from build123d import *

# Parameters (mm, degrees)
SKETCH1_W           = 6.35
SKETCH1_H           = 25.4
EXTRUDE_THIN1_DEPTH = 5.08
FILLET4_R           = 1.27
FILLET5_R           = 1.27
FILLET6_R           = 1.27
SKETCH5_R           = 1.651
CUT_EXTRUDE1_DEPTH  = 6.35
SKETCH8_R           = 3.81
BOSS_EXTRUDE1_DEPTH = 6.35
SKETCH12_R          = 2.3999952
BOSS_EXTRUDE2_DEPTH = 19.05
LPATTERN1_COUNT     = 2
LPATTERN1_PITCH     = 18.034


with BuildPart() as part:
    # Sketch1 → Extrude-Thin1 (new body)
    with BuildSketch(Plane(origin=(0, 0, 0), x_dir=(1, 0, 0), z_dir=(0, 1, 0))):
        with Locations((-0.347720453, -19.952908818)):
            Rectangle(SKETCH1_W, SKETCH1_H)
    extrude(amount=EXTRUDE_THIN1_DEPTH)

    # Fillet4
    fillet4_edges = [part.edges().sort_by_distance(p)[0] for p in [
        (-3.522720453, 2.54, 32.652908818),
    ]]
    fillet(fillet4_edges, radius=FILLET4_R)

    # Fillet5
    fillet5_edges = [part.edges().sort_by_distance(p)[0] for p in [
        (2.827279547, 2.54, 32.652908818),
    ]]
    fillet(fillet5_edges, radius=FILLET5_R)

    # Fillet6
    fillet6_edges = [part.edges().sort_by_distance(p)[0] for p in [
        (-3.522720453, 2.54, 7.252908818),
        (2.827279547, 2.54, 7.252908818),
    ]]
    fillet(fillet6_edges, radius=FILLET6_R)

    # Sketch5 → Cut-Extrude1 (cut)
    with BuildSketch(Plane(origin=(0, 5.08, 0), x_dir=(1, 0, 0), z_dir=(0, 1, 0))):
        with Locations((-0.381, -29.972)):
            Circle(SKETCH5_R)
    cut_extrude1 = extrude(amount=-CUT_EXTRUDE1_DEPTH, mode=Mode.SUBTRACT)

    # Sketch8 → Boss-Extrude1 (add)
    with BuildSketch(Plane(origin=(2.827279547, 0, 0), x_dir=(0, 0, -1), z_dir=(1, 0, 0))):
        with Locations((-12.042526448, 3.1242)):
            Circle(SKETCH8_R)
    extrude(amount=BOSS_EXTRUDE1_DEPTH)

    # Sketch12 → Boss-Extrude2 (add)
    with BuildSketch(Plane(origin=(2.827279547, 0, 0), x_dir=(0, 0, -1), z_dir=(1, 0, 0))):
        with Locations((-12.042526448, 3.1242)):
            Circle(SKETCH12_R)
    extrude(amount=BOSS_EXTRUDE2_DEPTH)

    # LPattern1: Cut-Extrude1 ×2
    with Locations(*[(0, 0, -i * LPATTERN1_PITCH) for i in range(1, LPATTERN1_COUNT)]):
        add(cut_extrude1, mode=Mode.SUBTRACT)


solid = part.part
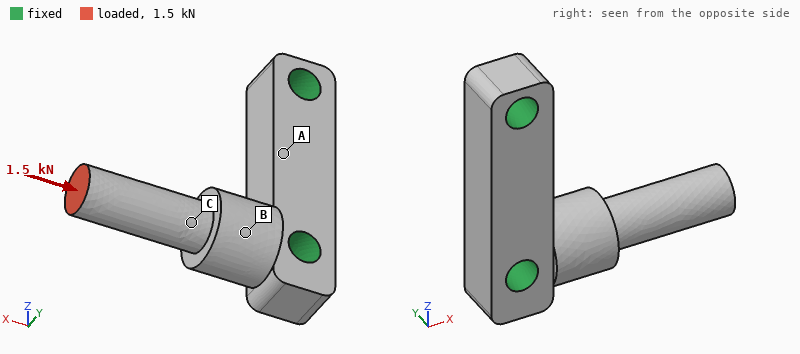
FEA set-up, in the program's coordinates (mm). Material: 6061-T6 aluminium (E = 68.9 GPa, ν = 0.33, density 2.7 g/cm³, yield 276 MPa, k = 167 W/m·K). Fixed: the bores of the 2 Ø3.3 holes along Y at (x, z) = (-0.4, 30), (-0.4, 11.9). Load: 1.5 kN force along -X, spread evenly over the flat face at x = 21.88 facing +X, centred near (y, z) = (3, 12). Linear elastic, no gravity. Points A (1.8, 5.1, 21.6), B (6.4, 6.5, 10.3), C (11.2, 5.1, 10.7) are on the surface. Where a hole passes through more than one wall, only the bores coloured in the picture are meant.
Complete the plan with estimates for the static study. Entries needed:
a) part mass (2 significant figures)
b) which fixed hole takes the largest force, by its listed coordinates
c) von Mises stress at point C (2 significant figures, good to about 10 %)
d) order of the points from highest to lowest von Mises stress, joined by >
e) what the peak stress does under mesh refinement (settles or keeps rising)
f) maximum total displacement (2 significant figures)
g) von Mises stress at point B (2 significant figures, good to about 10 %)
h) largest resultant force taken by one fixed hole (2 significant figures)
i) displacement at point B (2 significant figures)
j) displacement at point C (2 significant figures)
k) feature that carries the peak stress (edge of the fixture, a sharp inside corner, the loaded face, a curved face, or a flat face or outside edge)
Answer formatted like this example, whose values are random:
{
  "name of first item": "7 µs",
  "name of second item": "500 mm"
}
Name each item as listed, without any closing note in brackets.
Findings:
{
  "part mass": "3.4 g",
  "which fixed hole takes the largest force, by its listed coordinates": "(-0.4, 11.9)",
  "von Mises stress at point C": "81 MPa",
  "order of the points from highest to lowest von Mises stress, joined by >": "C > B > A",
  "what the peak stress does under mesh refinement": "keeps rising",
  "maximum total displacement": "25 µm",
  "von Mises stress at point B": "22 MPa",
  "largest resultant force taken by one fixed hole": "1.5 kN",
  "displacement at point B": "6.5 µm",
  "displacement at point C": "11 µm",
  "feature that carries the peak stress": "edge of the fixture"
}
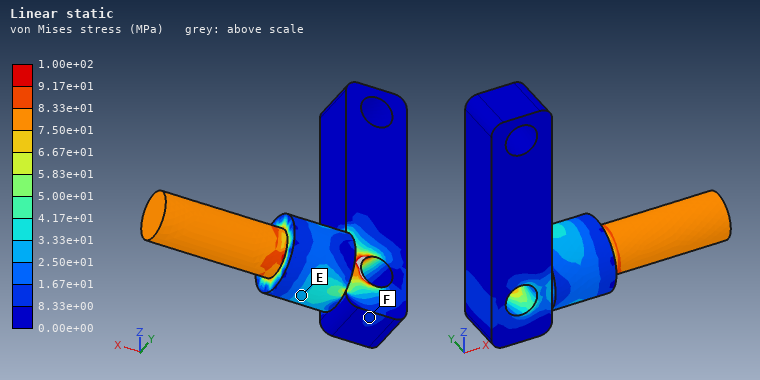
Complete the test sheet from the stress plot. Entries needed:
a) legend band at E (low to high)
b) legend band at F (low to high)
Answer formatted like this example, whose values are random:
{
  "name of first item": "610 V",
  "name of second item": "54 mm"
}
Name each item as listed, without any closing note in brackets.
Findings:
{
  "legend band at E": "2.50e+01 to 3.33e+01 MPa",
  "legend band at F": "8.33e+00 to 1.67e+01 MPa"
}
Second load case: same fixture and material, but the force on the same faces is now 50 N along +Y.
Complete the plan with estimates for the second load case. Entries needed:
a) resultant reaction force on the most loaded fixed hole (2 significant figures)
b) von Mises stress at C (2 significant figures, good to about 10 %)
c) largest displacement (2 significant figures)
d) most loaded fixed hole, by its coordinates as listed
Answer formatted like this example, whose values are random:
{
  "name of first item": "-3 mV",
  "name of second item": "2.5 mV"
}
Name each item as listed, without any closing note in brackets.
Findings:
{
  "resultant reaction force on the most loaded fixed hole": "55 N",
  "von Mises stress at C": "41 MPa",
  "largest displacement": "43 µm",
  "most loaded fixed hole, by its coordinates as listed": "(-0.4, 11.9)"
}
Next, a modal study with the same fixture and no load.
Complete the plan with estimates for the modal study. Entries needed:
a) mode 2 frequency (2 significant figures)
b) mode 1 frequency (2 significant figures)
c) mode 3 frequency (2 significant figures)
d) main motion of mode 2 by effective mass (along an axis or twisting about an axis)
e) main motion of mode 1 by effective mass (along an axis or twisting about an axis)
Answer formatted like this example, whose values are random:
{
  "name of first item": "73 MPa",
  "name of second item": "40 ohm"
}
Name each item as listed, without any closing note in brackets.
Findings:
{
  "mode 2 frequency": "13 kHz",
  "mode 1 frequency": "12 kHz",
  "mode 3 frequency": "41 kHz",
  "main motion of mode 2 by effective mass": "along Z",
  "main motion of mode 1 by effective mass": "along Y"
}
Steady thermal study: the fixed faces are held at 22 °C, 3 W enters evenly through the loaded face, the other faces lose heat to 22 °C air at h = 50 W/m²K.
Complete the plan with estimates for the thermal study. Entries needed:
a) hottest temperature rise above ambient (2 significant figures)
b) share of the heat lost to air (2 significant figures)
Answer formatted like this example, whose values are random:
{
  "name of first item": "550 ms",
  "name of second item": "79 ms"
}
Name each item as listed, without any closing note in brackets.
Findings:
{
  "hottest temperature rise above ambient": "16 K",
  "share of the heat lost to air": "4.1 %"
}
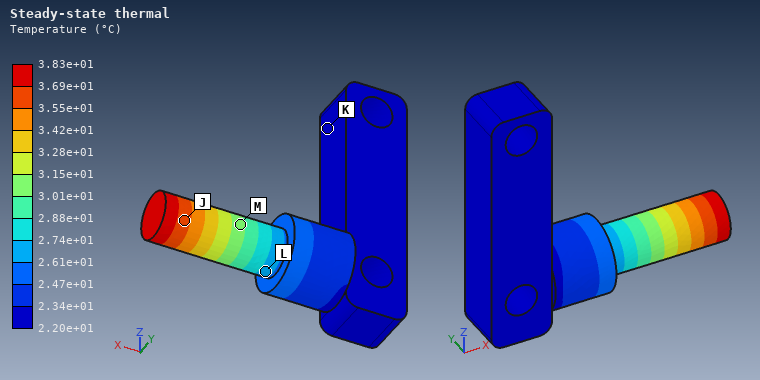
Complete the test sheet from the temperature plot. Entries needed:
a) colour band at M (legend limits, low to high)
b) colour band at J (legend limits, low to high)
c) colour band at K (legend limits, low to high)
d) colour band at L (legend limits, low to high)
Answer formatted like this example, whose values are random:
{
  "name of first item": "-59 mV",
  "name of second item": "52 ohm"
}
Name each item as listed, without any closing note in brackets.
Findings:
{
  "colour band at M": "3.01e+01 to 3.15e+01 °C",
  "colour band at J": "3.55e+01 to 3.69e+01 °C",
  "colour band at K": "2.20e+01 to 2.34e+01 °C",
  "colour band at L": "2.61e+01 to 2.74e+01 °C"
}
